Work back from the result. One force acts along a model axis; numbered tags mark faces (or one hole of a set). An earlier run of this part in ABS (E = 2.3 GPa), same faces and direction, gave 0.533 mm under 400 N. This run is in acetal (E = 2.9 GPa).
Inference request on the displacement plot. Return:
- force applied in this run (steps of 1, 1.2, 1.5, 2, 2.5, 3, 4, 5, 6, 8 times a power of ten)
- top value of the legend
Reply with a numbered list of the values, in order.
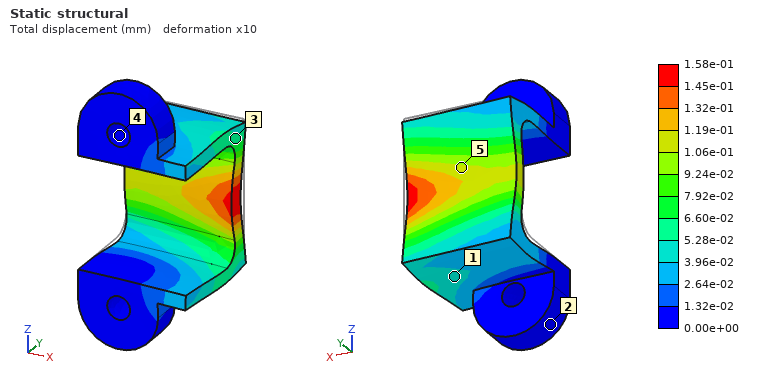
1. 150 N
2. 1.58e-01 mm
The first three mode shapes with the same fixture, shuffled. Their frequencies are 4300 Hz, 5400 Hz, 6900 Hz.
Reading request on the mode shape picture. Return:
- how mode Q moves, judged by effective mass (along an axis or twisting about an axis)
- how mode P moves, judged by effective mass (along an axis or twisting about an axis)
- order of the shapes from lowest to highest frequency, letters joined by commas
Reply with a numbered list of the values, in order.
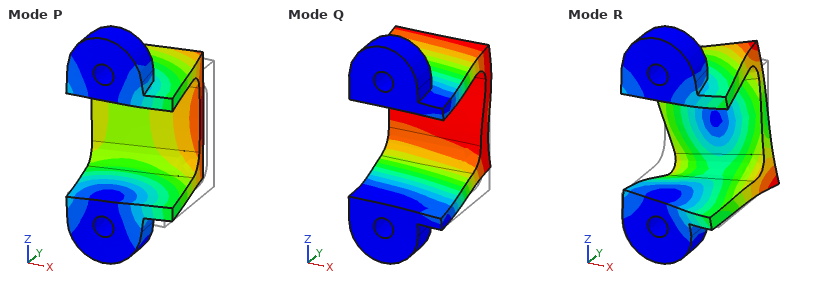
1. along Z
2. along X
3. Q, P, R
